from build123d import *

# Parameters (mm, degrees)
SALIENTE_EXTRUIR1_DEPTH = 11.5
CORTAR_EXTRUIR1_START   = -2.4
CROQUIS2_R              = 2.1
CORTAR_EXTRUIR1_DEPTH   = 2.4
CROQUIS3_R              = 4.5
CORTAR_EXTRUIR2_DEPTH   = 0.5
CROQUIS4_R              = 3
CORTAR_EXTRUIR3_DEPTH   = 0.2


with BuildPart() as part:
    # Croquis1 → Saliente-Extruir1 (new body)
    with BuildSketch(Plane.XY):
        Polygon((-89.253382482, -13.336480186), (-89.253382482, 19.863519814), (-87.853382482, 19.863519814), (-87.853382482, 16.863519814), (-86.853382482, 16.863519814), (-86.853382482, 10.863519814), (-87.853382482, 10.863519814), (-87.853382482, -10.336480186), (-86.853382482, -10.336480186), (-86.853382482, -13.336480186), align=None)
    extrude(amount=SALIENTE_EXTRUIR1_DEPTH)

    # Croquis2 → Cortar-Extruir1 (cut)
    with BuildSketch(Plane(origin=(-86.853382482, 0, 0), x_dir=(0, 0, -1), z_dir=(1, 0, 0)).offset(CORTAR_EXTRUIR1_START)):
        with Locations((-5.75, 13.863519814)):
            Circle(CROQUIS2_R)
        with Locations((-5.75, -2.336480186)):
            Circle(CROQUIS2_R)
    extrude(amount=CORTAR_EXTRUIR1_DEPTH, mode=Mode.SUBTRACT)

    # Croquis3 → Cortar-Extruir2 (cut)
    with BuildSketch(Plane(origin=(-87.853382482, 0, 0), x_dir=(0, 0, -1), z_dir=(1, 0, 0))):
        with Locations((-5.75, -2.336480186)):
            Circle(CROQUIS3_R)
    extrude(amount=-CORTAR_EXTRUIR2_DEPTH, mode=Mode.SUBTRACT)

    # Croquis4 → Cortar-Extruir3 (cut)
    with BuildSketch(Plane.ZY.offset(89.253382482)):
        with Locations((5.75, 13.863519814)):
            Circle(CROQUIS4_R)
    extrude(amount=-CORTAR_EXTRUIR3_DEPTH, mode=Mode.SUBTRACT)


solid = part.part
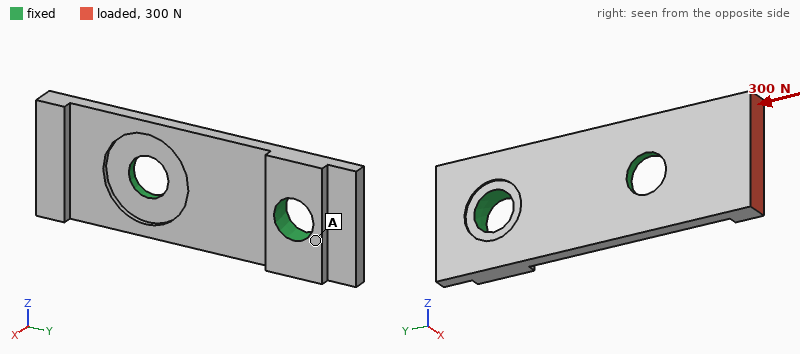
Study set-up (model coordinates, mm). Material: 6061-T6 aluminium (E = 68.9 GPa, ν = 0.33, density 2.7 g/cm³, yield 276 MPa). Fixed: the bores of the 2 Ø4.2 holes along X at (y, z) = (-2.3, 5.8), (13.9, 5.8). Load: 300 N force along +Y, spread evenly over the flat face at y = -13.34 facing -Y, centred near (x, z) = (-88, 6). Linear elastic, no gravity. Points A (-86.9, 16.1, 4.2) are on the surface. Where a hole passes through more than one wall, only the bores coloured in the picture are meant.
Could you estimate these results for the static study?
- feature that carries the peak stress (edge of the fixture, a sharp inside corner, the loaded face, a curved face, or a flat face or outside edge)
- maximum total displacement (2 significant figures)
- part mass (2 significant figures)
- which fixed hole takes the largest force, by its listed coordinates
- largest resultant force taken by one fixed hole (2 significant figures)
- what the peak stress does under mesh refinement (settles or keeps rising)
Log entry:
edge of the fixture
79 µm
1.5 g
(-2.3, 5.8)
250 N
keeps rising
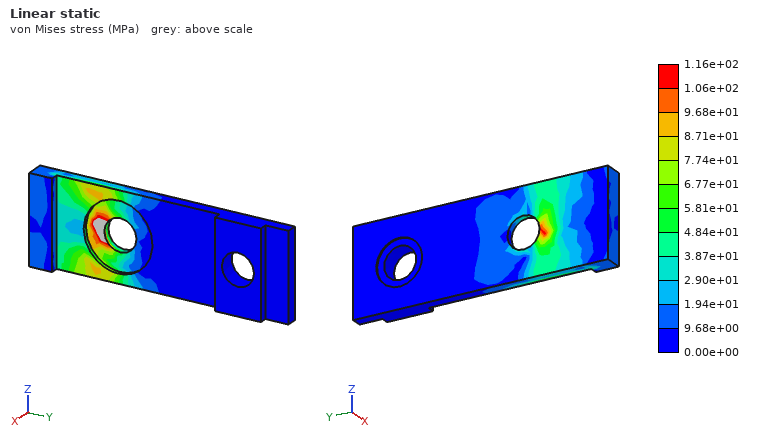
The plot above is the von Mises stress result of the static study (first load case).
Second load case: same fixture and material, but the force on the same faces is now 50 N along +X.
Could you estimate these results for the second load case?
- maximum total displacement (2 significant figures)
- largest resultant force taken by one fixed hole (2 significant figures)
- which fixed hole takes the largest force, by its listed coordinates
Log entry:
0.15 mm
62 N
(-2.3, 5.8)
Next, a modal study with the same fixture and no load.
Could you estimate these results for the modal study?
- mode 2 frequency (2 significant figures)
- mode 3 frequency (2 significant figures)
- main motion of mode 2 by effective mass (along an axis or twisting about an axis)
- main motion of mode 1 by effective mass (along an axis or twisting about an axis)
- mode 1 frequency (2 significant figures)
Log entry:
14 kHz
31 kHz
twisting about Y
along X
6900 Hz
